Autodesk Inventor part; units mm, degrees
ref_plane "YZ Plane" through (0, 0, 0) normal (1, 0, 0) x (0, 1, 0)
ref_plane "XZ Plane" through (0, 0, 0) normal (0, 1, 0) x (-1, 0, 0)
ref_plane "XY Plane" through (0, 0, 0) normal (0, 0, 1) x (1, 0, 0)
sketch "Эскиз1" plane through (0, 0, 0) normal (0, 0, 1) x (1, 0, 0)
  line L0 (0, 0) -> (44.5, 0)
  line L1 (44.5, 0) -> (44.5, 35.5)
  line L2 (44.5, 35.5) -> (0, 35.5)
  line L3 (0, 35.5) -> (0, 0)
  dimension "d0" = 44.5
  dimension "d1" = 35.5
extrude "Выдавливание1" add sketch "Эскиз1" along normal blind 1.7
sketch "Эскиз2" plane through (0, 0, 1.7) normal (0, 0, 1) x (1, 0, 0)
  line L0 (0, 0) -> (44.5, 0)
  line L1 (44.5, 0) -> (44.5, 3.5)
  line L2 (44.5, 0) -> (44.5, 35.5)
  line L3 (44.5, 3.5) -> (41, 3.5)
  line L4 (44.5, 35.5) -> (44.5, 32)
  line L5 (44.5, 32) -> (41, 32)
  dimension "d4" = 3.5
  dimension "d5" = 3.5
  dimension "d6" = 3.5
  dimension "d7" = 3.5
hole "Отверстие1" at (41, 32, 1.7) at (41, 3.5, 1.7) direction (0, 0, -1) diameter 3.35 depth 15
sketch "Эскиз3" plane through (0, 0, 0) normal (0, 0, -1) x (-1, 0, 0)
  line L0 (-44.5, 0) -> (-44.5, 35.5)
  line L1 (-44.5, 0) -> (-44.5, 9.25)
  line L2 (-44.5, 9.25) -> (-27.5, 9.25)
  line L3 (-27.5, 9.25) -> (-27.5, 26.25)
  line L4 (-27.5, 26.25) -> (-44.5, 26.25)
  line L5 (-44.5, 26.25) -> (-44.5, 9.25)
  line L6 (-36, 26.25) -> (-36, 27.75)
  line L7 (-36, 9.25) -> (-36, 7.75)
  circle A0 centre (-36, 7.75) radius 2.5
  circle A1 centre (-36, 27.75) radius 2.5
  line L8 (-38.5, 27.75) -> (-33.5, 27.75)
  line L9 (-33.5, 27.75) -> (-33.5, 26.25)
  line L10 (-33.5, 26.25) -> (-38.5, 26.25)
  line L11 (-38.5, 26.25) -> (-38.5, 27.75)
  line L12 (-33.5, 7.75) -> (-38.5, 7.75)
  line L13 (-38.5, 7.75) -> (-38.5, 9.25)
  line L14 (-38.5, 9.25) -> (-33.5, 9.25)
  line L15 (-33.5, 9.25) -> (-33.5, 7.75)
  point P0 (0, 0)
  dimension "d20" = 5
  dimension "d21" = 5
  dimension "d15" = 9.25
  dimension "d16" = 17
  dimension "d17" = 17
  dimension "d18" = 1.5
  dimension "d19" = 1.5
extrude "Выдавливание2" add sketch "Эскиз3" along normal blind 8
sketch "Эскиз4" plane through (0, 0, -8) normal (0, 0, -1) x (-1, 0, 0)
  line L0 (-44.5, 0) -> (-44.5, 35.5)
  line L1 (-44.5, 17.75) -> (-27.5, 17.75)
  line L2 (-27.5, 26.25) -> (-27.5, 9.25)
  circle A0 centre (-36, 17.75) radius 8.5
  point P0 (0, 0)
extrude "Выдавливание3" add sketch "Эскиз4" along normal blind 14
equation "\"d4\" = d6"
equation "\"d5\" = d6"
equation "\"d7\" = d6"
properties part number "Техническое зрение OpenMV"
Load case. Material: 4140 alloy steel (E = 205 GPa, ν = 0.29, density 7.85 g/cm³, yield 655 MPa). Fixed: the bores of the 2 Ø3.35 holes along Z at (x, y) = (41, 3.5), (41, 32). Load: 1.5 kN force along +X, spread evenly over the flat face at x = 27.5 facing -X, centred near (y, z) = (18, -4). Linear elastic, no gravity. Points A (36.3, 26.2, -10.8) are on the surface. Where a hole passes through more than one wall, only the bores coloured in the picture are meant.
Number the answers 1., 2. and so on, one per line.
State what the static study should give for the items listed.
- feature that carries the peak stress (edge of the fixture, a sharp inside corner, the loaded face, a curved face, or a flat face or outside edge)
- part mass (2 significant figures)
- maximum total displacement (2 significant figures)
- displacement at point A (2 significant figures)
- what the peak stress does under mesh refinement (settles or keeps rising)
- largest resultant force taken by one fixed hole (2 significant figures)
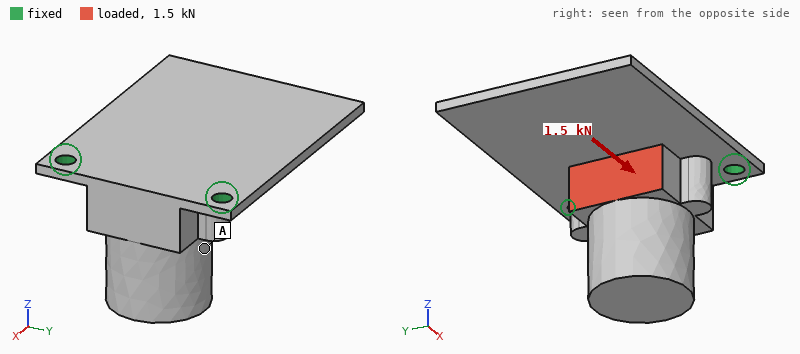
1. edge of the fixture
2. 66 g
3. 0.30 mm
4. 0.091 mm
5. keeps rising
6. 810 N
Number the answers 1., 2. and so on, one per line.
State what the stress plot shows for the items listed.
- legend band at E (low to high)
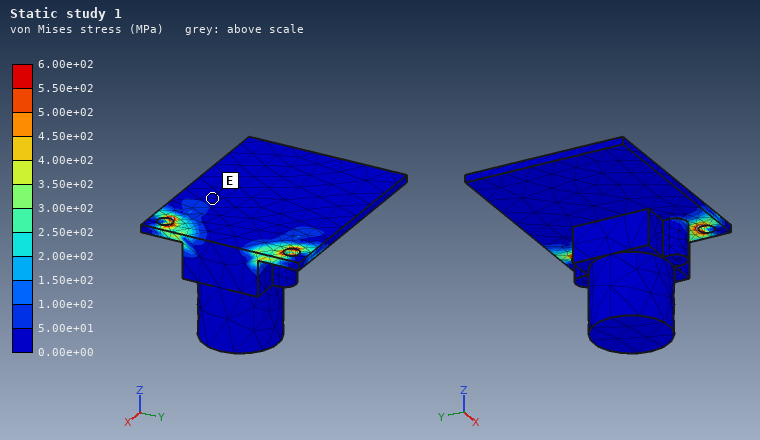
1. 0.00e+00 to 5.00e+01 MPa
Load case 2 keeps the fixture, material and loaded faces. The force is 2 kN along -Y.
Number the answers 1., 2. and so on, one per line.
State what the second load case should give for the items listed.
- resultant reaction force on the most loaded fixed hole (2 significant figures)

1. 1.4 kN
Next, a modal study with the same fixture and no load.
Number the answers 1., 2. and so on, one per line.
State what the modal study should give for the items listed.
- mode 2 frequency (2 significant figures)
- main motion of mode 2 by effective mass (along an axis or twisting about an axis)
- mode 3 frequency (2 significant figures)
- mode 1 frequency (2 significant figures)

1. 2600 Hz
2. along X
3. 3100 Hz
4. 1000 Hz
